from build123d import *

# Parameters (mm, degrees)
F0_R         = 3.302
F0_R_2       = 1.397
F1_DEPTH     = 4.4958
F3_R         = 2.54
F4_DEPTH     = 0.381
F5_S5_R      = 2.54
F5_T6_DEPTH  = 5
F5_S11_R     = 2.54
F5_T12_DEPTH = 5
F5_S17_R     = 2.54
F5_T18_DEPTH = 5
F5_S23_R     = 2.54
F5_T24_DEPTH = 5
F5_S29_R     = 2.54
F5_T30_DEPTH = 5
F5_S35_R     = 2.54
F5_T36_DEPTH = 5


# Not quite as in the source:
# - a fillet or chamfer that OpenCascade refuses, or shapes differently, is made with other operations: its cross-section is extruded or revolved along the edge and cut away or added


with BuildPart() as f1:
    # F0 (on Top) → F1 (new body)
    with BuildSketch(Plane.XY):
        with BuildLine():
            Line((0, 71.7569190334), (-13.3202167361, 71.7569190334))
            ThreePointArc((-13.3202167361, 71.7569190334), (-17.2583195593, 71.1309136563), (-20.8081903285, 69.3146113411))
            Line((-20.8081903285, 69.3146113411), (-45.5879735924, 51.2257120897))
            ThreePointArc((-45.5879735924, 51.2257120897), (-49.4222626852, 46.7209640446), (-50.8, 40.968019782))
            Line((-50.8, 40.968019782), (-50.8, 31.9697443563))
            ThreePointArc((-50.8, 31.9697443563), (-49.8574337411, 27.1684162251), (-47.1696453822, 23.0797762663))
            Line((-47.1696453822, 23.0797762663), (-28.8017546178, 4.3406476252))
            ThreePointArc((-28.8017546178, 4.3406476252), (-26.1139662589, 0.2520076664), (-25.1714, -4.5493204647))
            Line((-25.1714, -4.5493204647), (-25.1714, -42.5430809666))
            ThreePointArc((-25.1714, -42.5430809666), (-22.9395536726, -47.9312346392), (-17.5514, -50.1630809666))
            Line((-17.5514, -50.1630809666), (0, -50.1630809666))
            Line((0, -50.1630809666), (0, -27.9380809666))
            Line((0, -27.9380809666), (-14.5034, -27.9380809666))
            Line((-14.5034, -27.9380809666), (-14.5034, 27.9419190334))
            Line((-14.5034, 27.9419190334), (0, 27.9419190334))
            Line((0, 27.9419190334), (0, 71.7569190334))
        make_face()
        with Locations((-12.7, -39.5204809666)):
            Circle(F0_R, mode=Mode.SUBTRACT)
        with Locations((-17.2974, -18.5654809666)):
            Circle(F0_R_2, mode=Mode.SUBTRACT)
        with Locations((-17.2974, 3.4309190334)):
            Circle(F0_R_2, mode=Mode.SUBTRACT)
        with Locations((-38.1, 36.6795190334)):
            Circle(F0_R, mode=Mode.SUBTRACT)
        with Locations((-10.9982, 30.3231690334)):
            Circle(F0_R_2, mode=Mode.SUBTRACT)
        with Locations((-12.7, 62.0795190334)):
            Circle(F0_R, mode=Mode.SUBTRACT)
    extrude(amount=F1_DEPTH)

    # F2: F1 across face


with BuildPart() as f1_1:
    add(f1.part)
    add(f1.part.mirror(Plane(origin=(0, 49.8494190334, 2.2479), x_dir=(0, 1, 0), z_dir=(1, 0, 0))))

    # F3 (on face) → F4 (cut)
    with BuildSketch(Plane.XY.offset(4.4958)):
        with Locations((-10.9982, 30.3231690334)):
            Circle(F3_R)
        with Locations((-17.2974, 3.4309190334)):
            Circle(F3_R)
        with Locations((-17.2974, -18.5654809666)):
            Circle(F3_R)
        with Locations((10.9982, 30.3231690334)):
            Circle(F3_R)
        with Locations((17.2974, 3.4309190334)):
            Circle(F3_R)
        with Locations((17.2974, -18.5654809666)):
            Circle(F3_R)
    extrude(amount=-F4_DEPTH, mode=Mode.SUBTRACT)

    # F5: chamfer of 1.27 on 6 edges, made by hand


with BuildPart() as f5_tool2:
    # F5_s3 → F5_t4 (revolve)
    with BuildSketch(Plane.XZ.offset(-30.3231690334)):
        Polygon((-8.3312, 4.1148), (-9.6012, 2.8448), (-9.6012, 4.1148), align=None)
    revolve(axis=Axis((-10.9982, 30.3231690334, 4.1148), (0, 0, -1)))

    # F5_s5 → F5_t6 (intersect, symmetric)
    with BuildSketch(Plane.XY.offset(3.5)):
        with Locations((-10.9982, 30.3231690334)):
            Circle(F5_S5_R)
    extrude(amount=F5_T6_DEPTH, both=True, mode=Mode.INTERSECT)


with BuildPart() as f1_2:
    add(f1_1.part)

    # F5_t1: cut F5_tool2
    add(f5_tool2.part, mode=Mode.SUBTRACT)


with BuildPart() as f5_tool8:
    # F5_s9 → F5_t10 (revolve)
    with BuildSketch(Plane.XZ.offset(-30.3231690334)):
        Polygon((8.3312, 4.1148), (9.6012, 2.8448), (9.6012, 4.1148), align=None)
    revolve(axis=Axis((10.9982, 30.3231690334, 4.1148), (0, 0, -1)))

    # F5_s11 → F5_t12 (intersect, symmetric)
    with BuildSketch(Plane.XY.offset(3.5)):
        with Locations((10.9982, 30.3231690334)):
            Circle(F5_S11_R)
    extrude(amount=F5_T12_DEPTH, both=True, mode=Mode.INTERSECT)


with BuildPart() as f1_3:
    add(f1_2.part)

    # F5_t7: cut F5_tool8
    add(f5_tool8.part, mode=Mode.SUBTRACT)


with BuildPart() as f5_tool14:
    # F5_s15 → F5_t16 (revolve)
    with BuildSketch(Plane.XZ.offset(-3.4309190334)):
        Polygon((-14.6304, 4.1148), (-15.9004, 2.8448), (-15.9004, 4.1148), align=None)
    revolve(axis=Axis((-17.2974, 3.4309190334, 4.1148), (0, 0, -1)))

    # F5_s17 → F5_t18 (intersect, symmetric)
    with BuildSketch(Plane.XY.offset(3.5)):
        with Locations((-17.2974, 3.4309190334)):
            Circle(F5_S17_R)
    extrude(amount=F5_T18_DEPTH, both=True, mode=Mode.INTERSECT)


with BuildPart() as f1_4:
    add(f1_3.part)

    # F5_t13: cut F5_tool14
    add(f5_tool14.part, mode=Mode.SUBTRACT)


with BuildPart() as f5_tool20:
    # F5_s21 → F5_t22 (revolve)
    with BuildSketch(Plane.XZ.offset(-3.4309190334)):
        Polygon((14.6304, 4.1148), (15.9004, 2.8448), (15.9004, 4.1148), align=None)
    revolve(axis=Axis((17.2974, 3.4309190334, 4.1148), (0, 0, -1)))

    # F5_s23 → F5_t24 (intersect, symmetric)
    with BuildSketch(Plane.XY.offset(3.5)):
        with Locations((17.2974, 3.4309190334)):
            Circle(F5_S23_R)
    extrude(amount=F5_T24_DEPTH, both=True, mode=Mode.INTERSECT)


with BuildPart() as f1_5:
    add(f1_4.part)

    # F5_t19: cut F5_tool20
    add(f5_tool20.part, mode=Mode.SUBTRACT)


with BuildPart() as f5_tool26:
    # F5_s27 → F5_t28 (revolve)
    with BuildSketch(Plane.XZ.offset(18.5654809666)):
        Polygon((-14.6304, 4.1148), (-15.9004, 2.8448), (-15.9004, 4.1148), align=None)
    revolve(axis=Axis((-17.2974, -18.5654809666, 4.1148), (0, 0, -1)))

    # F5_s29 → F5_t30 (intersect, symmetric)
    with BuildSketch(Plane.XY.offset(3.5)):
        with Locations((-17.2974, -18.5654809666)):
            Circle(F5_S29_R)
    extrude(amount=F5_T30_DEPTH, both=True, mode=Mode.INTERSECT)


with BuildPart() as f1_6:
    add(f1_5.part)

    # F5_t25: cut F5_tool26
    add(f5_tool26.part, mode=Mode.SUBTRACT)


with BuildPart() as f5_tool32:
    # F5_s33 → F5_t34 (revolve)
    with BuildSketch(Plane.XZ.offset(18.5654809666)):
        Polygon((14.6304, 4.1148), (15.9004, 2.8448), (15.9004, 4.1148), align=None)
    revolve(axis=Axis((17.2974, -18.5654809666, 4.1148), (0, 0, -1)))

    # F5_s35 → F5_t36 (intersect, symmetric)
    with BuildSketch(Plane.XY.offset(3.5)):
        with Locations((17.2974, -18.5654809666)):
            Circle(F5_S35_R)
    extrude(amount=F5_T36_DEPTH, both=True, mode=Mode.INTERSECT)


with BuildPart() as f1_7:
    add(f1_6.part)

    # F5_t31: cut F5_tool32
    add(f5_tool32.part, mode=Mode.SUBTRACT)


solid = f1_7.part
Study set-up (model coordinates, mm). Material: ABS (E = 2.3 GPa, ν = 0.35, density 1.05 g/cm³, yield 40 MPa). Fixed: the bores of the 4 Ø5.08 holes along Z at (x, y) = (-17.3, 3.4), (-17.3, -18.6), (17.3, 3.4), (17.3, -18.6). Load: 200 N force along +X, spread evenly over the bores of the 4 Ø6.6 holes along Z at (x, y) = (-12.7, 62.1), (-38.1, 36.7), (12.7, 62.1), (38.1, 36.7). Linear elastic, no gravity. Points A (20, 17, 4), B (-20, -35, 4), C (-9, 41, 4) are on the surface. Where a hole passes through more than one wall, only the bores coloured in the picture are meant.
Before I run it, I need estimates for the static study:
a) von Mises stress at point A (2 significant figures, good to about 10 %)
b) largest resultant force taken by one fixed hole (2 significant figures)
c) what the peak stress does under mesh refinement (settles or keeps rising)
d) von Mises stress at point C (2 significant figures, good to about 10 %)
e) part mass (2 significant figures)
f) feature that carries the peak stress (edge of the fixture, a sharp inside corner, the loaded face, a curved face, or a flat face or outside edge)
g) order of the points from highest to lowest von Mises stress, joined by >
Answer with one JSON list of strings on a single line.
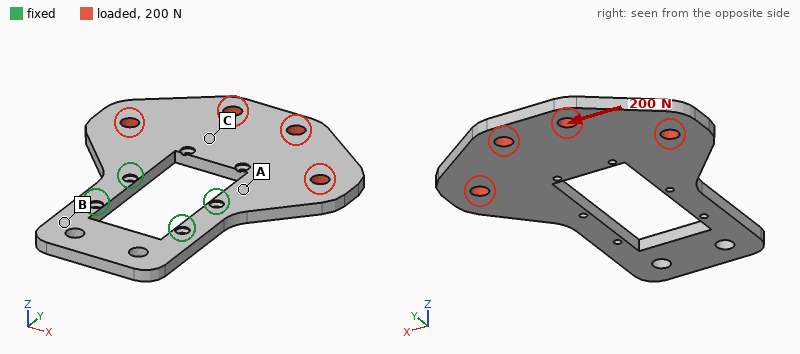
["4.3 MPa", "170 N", "keeps rising", "2.5 MPa", "30 g", "edge of the fixture", "A > C > B"]
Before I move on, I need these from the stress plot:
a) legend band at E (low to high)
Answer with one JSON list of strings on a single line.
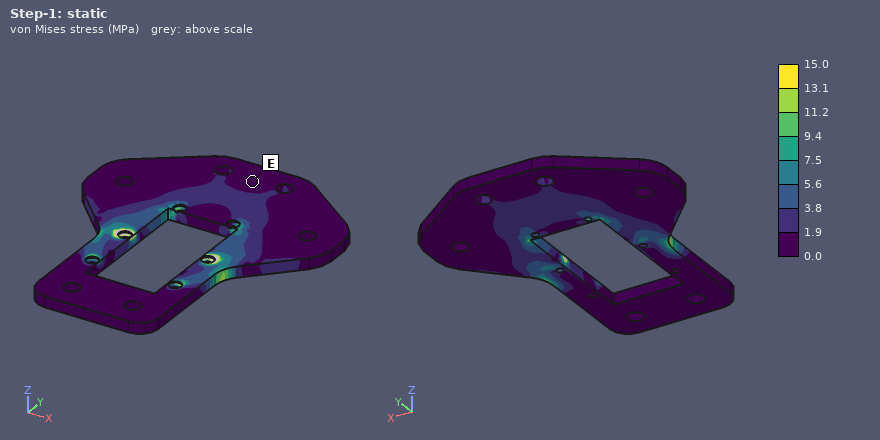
["0.0 to 1.9 MPa"]
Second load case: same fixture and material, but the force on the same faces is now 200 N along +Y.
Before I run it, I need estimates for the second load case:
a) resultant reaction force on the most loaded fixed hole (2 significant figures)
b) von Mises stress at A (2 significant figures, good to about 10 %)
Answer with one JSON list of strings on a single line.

["71 N", "1.5 MPa"]
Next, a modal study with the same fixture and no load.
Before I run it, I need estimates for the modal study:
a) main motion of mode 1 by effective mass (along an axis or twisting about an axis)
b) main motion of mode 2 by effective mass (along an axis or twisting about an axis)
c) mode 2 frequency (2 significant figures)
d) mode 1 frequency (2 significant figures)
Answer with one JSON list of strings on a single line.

["along Z", "twisting about Y", "330 Hz", "160 Hz"]
